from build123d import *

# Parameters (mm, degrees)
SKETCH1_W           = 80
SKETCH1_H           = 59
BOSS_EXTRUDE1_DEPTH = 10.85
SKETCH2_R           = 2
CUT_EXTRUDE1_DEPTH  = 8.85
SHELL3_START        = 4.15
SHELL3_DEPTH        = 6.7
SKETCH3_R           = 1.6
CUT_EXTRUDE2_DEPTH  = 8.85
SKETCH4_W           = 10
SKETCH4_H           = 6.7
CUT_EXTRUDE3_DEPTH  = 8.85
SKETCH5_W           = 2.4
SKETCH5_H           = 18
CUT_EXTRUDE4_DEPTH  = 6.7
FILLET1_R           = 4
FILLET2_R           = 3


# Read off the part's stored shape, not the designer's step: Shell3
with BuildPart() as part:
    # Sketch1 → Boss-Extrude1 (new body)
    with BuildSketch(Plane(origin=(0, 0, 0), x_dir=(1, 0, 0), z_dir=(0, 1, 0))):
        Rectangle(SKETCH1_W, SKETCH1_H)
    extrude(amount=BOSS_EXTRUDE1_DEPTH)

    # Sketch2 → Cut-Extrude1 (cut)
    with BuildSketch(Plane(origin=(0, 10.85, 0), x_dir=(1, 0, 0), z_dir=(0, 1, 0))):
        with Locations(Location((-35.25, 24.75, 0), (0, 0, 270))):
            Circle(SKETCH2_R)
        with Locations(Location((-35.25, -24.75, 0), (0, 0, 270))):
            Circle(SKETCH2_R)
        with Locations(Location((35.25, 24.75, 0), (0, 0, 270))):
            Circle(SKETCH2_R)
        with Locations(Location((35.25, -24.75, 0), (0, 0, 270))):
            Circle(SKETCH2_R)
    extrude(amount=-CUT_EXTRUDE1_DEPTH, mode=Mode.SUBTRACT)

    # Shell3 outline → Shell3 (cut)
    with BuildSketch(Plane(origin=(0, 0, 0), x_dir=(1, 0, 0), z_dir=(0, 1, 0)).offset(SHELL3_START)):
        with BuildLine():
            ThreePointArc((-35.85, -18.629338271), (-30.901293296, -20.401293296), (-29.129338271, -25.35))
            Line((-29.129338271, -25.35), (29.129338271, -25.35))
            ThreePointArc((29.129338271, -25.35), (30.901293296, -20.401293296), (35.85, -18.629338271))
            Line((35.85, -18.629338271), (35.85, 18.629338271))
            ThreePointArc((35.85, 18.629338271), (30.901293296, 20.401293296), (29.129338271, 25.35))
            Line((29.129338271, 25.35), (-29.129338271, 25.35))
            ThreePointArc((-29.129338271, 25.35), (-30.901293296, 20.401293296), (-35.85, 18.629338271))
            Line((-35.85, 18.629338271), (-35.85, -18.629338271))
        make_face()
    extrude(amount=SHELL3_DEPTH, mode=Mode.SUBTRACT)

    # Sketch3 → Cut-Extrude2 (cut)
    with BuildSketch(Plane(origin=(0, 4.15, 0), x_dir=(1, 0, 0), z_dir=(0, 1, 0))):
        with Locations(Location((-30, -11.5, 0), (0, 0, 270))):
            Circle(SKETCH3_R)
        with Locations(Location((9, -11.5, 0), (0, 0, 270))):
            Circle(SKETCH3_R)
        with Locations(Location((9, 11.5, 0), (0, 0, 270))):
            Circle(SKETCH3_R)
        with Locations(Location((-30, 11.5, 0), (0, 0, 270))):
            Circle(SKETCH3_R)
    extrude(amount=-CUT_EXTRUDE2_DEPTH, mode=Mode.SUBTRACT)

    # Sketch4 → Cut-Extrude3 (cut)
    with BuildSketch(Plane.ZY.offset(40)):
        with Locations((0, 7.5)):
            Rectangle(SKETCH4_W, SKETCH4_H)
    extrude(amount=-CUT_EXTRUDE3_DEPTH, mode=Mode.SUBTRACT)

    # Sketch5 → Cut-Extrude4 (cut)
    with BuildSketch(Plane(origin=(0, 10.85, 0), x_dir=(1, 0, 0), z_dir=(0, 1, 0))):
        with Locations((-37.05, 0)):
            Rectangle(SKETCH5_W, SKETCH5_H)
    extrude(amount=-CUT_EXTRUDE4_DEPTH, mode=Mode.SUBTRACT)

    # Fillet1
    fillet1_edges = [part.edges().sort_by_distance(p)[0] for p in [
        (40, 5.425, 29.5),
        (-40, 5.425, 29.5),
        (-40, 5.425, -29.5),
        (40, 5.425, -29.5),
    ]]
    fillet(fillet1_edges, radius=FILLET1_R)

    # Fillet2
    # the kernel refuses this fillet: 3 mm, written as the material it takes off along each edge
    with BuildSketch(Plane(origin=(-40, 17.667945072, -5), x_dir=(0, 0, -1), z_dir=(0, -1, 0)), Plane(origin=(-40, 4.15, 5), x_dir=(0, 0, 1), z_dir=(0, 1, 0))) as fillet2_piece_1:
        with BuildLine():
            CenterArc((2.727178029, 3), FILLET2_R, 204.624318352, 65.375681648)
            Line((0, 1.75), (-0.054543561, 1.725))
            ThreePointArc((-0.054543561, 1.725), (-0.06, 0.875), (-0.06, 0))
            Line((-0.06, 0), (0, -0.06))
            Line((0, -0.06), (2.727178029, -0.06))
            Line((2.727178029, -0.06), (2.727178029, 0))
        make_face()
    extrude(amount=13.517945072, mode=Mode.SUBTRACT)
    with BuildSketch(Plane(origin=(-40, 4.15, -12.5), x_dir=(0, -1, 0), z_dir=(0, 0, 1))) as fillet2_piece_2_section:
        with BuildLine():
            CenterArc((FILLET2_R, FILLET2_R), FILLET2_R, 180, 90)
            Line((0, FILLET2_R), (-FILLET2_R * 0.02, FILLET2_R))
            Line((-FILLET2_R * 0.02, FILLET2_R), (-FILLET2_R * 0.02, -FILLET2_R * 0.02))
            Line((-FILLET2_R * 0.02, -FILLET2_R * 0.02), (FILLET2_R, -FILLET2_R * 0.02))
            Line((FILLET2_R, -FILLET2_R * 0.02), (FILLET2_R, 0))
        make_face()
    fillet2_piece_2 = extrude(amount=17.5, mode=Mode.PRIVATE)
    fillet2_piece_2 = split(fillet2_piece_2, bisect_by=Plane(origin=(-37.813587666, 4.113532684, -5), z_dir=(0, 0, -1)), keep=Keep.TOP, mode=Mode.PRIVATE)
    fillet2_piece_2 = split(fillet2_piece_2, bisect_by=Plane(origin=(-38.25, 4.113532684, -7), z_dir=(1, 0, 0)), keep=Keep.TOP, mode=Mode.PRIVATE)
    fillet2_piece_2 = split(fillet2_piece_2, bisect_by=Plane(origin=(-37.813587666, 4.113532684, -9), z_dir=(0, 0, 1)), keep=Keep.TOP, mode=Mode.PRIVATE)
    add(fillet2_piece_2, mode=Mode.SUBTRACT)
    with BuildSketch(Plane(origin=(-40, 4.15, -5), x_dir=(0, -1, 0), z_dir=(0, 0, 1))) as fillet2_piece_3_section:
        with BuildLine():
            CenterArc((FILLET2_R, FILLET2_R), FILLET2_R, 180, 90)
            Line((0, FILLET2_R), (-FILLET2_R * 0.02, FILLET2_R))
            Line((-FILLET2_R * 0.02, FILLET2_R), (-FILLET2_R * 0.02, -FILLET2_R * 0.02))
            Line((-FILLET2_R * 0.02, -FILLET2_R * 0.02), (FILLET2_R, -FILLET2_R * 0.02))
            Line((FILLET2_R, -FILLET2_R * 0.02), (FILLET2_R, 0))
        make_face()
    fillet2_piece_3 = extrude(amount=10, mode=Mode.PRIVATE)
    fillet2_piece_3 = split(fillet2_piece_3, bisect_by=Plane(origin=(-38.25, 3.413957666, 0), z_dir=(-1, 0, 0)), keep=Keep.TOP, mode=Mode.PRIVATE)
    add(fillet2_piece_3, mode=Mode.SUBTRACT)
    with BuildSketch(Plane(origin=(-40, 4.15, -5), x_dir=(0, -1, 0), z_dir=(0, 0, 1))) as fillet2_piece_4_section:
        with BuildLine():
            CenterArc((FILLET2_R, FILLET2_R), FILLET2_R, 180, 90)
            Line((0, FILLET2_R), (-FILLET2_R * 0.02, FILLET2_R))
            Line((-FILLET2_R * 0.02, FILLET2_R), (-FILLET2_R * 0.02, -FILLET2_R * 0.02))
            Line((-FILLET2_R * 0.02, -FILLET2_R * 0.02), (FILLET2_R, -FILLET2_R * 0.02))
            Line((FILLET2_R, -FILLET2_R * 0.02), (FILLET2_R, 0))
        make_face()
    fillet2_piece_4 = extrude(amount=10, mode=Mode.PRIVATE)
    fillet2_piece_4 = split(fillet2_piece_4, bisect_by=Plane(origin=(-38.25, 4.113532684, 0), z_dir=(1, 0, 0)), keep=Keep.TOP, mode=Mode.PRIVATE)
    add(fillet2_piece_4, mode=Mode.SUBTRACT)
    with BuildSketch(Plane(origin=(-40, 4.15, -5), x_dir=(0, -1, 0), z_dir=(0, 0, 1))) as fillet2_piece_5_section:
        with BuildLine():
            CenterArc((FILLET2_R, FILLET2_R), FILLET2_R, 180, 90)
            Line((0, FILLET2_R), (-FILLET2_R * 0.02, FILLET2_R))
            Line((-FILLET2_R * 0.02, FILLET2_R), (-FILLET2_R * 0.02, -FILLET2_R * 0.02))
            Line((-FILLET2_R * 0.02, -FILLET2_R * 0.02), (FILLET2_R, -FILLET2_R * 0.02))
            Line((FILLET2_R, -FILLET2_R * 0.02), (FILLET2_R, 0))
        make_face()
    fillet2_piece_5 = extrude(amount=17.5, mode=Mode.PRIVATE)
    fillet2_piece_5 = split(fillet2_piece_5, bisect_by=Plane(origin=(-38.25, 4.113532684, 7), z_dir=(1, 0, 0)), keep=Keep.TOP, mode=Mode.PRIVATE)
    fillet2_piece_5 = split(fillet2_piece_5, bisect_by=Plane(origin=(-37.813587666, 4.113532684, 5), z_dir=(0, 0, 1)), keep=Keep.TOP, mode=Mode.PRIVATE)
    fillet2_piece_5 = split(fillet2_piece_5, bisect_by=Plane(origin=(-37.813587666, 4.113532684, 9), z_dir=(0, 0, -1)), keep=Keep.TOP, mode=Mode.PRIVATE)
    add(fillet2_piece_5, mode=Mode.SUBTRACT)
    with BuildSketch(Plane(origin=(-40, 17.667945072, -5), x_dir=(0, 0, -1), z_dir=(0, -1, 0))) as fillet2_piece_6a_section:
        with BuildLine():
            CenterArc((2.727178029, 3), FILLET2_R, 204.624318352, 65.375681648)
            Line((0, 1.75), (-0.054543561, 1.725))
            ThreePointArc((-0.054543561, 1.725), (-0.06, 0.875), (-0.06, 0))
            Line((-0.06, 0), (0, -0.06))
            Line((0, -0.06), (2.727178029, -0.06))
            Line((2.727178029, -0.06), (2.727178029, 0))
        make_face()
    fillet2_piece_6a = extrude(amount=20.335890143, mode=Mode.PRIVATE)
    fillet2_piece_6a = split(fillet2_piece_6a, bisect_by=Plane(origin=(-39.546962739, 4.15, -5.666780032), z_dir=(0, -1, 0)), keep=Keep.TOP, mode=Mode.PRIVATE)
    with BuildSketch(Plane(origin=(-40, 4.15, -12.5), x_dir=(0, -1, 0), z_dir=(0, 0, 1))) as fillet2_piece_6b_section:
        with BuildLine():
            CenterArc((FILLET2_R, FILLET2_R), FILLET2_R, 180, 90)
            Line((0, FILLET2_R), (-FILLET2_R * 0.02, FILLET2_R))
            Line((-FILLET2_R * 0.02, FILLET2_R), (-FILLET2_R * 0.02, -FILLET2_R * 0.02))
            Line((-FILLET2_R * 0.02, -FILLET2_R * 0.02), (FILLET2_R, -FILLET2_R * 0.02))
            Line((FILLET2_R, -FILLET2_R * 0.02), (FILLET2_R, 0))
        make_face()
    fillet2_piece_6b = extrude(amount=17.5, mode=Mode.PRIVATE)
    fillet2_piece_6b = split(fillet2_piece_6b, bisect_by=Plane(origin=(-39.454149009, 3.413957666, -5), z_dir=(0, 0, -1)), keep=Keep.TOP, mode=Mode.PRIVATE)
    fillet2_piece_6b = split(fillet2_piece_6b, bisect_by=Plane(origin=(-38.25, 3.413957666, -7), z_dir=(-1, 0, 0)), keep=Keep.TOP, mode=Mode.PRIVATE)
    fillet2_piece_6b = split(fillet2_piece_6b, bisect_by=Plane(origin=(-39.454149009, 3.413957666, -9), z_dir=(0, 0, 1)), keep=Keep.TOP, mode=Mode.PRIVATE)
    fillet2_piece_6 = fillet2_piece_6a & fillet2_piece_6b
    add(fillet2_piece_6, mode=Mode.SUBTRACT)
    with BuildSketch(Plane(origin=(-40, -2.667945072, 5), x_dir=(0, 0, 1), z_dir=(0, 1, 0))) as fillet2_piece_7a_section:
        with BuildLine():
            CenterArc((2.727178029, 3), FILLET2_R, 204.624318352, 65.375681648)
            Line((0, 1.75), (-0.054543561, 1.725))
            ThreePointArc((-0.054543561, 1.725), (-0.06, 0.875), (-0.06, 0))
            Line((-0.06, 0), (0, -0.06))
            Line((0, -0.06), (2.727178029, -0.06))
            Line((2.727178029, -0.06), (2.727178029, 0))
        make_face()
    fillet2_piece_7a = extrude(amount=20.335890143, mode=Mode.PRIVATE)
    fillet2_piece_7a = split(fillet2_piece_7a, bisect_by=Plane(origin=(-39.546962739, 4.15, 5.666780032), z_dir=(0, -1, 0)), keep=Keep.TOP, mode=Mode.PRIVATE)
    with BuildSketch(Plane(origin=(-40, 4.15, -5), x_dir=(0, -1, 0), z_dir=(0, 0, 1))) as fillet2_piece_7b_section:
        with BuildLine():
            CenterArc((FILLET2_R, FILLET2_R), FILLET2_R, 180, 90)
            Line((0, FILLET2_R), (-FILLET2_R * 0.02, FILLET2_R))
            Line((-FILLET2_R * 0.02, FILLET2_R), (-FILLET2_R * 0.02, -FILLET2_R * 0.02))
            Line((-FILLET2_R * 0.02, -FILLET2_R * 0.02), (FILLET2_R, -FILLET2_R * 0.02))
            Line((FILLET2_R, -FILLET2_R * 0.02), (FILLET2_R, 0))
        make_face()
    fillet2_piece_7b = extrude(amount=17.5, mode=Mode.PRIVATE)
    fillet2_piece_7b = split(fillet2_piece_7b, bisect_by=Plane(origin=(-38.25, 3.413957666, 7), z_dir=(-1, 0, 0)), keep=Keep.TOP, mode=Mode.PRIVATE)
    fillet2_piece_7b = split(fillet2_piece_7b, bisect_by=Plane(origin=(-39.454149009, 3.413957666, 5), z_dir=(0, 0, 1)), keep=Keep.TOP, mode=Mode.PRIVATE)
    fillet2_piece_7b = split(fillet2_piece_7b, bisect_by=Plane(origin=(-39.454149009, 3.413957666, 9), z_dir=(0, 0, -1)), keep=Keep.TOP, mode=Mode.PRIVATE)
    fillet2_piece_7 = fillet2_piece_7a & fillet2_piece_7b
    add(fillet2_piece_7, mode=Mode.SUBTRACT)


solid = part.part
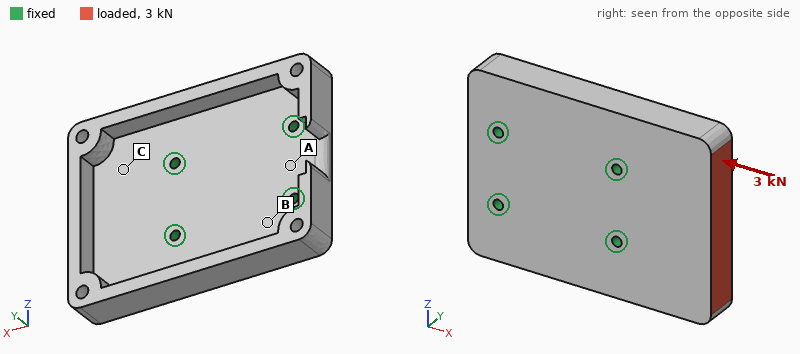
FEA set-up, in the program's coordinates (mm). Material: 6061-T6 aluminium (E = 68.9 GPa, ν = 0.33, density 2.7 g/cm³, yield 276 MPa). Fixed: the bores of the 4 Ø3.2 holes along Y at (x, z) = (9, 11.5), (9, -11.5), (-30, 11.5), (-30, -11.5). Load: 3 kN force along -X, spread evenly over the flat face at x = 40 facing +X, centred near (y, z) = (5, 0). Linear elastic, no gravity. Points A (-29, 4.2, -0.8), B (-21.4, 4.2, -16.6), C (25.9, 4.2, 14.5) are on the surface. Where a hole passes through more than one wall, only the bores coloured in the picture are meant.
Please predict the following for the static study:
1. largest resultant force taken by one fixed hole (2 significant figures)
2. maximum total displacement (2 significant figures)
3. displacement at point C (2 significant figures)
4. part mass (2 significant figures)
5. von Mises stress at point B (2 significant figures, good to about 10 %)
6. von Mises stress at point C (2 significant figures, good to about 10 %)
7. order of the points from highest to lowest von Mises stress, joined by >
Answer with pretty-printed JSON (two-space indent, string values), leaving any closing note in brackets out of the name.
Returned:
{
  "largest resultant force taken by one fixed hole": "1.2 kN",
  "maximum total displacement": "92 µm",
  "displacement at point C": "26 µm",
  "part mass": "72 g",
  "von Mises stress at point B": "9.4 MPa",
  "von Mises stress at point C": "27 MPa",
  "order of the points from highest to lowest von Mises stress, joined by >": "C > B > A"
}
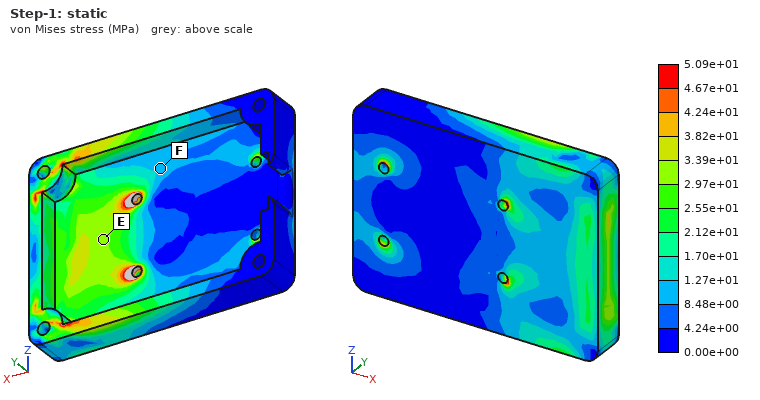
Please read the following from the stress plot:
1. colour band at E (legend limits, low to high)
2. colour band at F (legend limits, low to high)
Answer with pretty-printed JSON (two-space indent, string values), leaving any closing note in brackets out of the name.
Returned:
{
  "colour band at E": "2.97e+01 to 3.39e+01 MPa",
  "colour band at F": "8.48e+00 to 1.27e+01 MPa"
}
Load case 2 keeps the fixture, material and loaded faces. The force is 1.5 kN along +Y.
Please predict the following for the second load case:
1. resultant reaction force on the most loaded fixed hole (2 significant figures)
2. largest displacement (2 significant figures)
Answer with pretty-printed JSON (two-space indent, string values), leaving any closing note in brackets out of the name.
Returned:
{
  "resultant reaction force on the most loaded fixed hole": "1.3 kN",
  "largest displacement": "0.34 mm"
}
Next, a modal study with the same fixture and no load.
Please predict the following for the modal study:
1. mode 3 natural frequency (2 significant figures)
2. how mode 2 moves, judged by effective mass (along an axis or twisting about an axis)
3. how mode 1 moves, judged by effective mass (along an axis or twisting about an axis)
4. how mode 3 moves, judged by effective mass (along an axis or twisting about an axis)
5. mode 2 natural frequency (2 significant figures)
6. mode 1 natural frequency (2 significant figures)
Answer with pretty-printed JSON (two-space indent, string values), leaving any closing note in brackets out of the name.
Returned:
{
  "mode 3 natural frequency": "6300 Hz",
  "how mode 2 moves, judged by effective mass": "twisting about X",
  "how mode 1 moves, judged by effective mass": "along Y",
  "how mode 3 moves, judged by effective mass": "along Y",
  "mode 2 natural frequency": "3900 Hz",
  "mode 1 natural frequency": "3300 Hz"
}
